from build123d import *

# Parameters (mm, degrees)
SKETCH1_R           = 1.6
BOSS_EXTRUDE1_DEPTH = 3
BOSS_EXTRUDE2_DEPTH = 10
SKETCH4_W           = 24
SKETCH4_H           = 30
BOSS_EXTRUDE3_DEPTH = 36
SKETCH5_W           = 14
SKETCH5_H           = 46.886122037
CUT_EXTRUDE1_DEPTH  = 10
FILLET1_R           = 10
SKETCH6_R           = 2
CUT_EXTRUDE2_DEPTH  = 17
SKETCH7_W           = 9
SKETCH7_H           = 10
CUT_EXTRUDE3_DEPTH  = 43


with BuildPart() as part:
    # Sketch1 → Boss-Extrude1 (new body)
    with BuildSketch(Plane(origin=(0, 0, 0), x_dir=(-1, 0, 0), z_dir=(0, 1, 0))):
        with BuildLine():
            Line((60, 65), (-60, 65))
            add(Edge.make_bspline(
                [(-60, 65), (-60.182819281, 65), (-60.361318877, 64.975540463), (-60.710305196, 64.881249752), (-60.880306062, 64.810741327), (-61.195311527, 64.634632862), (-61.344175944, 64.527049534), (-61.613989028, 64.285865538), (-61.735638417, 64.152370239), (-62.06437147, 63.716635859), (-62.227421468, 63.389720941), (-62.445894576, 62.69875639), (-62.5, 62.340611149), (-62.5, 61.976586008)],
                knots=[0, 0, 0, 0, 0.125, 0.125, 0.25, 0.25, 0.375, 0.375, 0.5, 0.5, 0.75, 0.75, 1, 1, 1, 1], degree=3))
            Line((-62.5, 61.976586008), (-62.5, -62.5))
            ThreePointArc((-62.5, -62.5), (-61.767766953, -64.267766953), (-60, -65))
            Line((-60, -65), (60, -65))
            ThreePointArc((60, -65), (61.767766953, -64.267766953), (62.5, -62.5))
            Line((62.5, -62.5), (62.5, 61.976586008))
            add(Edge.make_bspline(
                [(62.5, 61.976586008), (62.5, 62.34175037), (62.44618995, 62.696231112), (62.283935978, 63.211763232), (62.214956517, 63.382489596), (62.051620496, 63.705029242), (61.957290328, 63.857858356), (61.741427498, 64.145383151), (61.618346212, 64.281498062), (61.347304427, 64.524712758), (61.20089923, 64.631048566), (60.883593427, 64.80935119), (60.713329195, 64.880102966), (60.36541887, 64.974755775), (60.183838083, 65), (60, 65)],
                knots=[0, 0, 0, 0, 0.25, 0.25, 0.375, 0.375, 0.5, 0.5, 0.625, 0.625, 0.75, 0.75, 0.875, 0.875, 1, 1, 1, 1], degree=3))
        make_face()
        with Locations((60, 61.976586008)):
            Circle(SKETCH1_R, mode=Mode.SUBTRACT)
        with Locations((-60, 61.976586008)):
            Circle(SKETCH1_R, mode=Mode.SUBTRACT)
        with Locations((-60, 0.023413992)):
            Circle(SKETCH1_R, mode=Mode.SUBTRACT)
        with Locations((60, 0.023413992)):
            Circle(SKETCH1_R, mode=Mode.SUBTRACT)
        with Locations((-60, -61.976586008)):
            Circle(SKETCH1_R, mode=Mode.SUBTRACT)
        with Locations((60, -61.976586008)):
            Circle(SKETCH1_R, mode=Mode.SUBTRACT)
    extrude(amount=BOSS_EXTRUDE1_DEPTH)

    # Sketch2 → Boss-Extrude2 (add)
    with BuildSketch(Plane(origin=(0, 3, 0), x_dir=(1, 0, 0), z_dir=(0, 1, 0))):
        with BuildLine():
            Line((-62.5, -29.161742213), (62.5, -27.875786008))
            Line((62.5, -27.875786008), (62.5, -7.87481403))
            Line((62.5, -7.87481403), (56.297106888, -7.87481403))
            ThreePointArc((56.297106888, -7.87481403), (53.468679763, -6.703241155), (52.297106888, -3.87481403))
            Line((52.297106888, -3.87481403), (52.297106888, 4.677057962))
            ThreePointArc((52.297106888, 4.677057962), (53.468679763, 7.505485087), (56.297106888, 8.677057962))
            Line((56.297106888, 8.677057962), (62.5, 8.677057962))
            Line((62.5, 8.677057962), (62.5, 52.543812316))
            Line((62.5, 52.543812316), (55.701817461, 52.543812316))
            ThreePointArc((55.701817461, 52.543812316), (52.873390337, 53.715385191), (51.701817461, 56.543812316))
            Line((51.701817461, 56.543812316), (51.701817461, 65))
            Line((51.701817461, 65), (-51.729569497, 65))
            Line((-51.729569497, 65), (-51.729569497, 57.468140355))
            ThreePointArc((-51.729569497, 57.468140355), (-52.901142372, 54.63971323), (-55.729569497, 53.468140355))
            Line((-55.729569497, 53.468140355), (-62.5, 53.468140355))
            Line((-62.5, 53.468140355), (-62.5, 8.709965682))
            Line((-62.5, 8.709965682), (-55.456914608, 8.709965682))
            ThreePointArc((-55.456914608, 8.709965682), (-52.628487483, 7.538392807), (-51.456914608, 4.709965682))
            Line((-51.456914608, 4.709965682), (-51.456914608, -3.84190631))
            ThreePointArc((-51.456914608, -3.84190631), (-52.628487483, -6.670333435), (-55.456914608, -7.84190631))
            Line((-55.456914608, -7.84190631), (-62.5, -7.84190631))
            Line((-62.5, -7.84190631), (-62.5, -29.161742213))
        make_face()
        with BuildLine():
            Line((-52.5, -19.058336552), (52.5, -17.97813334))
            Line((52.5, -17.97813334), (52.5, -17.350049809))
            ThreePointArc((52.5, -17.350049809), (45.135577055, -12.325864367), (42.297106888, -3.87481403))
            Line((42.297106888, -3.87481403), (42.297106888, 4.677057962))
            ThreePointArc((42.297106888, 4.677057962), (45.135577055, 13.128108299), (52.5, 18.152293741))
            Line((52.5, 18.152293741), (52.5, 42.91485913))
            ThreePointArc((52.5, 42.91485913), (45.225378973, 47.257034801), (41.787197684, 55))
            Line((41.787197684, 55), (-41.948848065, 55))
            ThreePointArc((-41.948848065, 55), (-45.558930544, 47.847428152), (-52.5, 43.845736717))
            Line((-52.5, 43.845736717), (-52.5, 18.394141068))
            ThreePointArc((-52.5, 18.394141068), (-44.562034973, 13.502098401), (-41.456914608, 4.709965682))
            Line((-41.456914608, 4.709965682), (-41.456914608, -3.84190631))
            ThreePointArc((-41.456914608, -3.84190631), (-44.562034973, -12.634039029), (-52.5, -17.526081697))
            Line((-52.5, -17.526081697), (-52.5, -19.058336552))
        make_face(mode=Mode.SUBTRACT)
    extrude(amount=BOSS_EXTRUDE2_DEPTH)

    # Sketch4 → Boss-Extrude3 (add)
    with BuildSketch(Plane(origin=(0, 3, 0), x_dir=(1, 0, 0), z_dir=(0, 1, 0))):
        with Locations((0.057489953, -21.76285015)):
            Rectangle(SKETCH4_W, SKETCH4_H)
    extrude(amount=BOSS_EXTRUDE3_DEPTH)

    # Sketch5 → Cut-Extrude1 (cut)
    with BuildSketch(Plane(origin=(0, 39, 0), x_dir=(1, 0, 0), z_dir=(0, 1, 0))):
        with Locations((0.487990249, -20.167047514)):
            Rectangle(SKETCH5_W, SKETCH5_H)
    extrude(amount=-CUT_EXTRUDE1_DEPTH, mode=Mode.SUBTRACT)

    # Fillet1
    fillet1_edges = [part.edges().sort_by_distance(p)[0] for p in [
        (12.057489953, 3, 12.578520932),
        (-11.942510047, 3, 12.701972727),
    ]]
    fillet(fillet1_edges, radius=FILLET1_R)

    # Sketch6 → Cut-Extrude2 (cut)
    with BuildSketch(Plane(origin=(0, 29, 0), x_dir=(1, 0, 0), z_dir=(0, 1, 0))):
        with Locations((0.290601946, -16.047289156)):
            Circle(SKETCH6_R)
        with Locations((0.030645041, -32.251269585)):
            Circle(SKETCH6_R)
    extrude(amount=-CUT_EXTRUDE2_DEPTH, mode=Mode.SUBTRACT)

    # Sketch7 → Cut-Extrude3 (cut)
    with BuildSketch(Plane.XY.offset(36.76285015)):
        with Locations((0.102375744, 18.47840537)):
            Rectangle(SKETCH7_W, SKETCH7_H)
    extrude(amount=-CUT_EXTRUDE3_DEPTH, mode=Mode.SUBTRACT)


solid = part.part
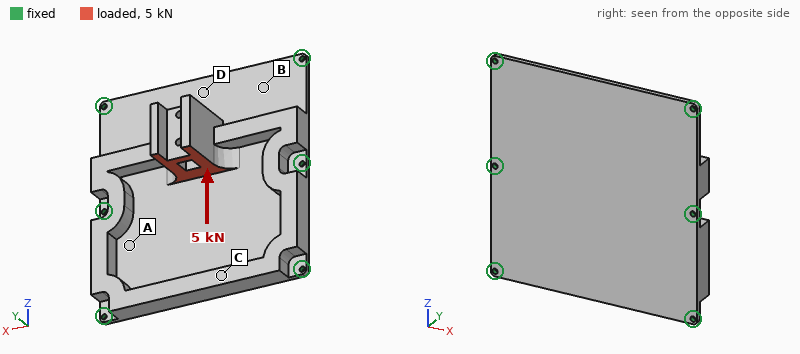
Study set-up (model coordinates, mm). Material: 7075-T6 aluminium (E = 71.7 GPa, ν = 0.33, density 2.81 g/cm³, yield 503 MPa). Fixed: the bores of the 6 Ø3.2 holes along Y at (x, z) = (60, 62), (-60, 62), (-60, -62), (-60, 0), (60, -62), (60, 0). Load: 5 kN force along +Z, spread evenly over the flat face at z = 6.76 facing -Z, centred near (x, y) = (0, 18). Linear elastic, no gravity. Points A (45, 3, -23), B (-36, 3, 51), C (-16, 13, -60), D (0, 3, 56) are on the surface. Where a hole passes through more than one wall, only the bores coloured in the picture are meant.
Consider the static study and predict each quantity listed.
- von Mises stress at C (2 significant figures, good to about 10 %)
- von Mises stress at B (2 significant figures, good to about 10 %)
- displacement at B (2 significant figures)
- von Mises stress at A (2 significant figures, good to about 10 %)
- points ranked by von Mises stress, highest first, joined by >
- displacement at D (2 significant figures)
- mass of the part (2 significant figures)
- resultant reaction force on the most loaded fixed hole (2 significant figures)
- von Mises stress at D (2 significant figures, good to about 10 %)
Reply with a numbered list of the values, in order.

1. 14 MPa
2. 67 MPa
3. 0.23 mm
4. 27 MPa
5. B > D > A > C
6. 0.51 mm
7. 300 g
8. 1.3 kN
9. 42 MPa
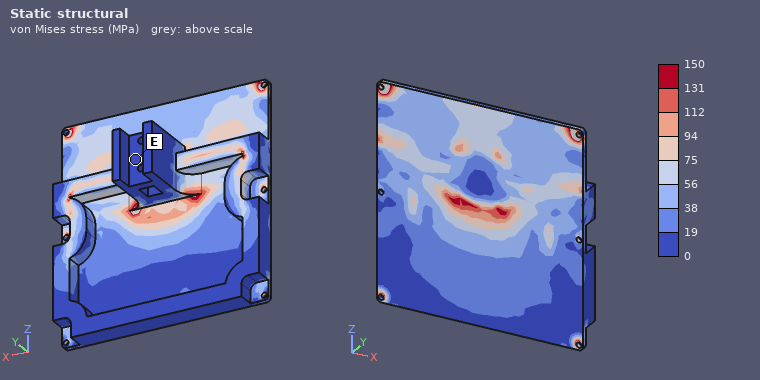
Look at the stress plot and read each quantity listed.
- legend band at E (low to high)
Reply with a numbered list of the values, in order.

1. 0 to 19 MPa
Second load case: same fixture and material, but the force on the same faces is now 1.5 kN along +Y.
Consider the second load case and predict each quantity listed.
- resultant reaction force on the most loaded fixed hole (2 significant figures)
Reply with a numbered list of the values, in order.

1. 1.1 kN
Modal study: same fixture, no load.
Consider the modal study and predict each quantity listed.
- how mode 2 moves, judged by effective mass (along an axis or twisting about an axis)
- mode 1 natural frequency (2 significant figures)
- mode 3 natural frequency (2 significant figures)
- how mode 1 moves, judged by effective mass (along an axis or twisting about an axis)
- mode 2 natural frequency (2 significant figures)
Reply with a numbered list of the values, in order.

1. along Y
2. 1300 Hz
3. 2700 Hz
4. along Y
5. 1900 Hz
